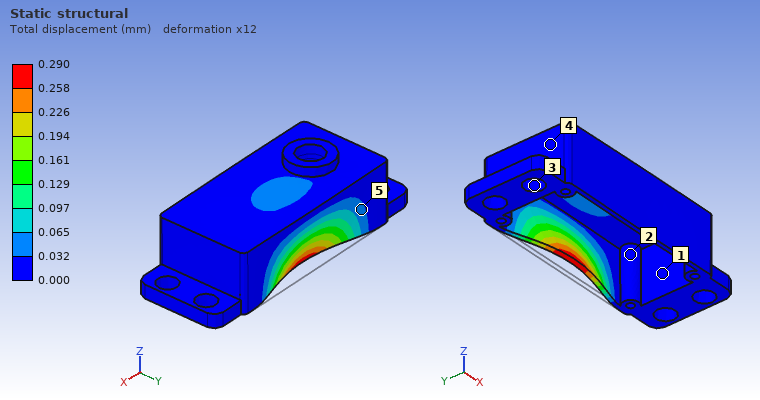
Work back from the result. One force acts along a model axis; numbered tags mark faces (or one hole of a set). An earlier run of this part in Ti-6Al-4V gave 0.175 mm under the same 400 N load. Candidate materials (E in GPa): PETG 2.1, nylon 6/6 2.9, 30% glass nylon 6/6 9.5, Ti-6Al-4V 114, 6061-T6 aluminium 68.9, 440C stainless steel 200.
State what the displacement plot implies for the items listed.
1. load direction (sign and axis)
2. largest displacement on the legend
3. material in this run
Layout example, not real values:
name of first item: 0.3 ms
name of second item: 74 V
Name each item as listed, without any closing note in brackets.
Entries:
load direction: -Y
largest displacement on the legend: 0.290 mm
material in this run: 6061-T6 aluminium
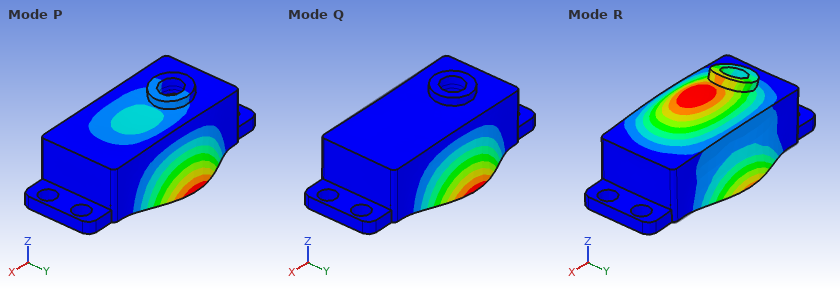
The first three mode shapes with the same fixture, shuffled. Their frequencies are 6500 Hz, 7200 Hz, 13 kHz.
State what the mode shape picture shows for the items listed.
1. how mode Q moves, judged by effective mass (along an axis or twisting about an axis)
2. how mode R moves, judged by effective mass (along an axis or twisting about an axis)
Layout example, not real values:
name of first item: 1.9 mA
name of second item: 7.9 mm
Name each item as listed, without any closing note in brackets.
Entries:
how mode Q moves, judged by effective mass: along Y
how mode R moves, judged by effective mass: along Z
